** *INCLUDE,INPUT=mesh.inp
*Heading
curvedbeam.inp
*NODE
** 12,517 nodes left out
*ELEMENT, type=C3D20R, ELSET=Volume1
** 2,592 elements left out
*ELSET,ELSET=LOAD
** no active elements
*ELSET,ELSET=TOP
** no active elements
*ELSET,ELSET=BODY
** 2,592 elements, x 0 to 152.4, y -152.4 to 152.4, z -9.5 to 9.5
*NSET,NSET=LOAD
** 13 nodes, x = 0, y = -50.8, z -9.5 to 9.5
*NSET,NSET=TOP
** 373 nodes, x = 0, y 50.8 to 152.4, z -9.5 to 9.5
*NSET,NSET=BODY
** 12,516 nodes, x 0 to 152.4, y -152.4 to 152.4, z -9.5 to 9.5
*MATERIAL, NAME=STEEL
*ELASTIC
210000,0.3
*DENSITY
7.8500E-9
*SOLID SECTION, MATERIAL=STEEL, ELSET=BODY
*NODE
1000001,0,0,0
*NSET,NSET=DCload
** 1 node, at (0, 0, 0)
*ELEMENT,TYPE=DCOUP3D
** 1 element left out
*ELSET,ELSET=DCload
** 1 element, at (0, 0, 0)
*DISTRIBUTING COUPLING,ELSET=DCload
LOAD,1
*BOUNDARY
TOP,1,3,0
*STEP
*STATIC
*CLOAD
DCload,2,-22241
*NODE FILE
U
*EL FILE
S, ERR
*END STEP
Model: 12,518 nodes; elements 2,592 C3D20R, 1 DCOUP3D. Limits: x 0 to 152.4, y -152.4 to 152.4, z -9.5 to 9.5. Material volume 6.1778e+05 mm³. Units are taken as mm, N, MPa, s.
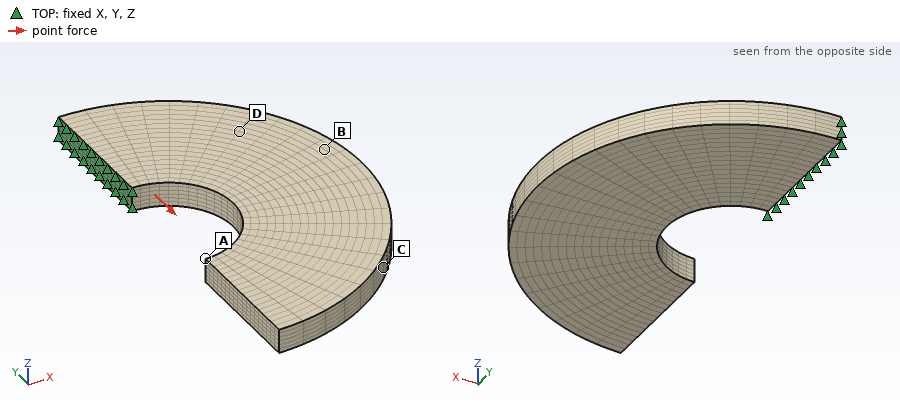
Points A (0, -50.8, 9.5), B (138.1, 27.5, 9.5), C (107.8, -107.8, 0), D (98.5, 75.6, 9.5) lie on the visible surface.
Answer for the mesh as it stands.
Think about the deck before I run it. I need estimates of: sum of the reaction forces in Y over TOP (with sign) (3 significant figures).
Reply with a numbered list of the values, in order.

1. 22200 N
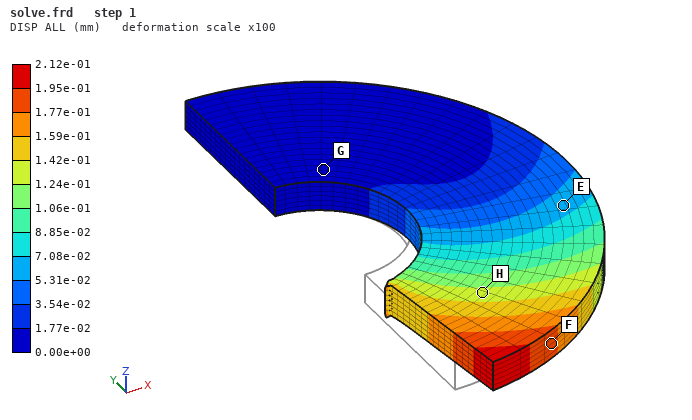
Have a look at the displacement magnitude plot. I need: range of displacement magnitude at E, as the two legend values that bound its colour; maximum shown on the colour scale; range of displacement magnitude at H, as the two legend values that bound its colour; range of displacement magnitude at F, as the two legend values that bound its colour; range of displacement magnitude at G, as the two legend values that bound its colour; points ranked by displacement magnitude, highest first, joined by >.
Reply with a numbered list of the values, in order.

1. 5.31e-02 to 7.08e-02 mm
2. 2.12e-01 mm
3. 1.24e-01 to 1.42e-01 mm
4. 1.77e-01 to 1.95e-01 mm
5. 0.00e+00 to 1.77e-02 mm
6. F > H > E > G
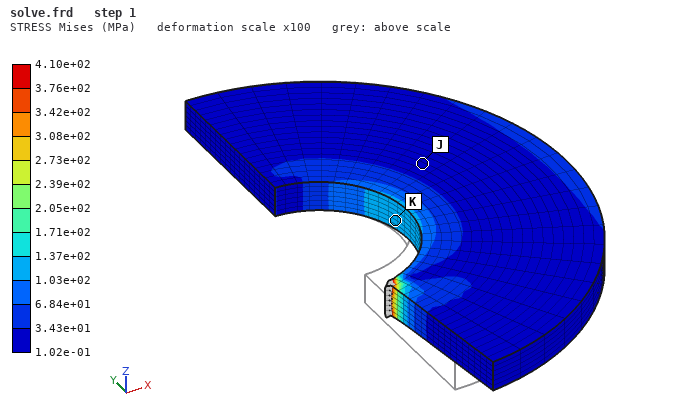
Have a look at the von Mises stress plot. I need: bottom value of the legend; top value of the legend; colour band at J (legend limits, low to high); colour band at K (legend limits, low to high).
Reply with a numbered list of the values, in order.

1. 1.02e-01 MPa
2. 4.10e+02 MPa
3. 1.02e-01 to 3.43e+01 MPa
4. 1.03e+02 to 1.37e+02 MPa
